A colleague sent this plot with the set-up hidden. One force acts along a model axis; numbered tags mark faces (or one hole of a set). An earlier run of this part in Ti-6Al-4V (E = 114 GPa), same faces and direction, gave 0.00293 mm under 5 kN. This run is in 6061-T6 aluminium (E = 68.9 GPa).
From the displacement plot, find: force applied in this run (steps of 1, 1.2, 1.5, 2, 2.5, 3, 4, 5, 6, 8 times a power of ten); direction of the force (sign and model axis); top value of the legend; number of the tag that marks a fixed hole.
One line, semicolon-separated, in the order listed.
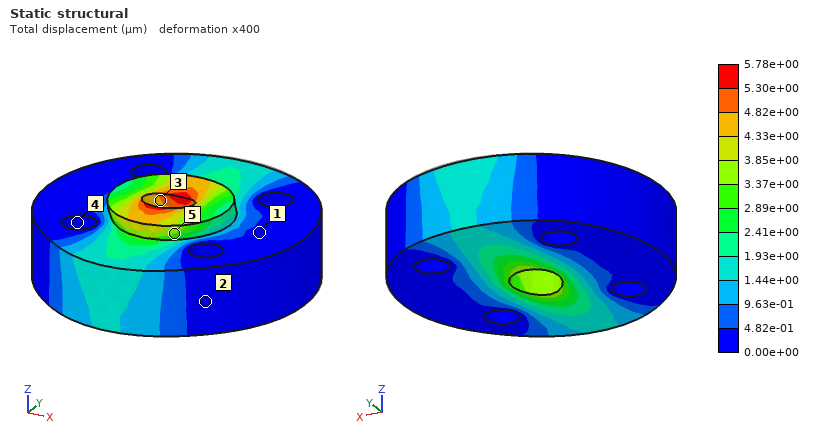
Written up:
6 kN; -Y; 5.78e+00 µm; 4
